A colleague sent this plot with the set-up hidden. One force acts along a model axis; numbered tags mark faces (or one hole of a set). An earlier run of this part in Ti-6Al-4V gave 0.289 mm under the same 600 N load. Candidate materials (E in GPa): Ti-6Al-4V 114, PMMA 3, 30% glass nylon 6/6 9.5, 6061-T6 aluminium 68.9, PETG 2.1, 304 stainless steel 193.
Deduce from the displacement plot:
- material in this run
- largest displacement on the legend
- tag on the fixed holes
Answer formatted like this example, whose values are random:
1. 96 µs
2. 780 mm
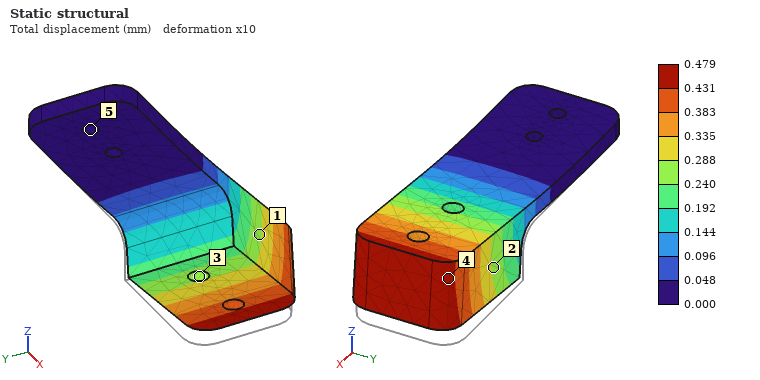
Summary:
1. 6061-T6 aluminium
2. 0.479 mm
3. 5
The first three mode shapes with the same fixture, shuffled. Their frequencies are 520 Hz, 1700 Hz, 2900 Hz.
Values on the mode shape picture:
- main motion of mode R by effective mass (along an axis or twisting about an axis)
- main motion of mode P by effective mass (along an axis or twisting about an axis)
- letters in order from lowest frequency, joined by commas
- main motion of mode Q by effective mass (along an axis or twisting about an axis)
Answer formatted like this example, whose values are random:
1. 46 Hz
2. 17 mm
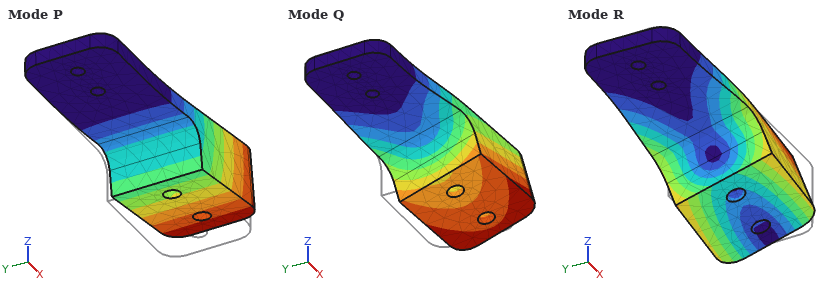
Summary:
1. along Y
2. along Z
3. P, Q, R
4. along Y
